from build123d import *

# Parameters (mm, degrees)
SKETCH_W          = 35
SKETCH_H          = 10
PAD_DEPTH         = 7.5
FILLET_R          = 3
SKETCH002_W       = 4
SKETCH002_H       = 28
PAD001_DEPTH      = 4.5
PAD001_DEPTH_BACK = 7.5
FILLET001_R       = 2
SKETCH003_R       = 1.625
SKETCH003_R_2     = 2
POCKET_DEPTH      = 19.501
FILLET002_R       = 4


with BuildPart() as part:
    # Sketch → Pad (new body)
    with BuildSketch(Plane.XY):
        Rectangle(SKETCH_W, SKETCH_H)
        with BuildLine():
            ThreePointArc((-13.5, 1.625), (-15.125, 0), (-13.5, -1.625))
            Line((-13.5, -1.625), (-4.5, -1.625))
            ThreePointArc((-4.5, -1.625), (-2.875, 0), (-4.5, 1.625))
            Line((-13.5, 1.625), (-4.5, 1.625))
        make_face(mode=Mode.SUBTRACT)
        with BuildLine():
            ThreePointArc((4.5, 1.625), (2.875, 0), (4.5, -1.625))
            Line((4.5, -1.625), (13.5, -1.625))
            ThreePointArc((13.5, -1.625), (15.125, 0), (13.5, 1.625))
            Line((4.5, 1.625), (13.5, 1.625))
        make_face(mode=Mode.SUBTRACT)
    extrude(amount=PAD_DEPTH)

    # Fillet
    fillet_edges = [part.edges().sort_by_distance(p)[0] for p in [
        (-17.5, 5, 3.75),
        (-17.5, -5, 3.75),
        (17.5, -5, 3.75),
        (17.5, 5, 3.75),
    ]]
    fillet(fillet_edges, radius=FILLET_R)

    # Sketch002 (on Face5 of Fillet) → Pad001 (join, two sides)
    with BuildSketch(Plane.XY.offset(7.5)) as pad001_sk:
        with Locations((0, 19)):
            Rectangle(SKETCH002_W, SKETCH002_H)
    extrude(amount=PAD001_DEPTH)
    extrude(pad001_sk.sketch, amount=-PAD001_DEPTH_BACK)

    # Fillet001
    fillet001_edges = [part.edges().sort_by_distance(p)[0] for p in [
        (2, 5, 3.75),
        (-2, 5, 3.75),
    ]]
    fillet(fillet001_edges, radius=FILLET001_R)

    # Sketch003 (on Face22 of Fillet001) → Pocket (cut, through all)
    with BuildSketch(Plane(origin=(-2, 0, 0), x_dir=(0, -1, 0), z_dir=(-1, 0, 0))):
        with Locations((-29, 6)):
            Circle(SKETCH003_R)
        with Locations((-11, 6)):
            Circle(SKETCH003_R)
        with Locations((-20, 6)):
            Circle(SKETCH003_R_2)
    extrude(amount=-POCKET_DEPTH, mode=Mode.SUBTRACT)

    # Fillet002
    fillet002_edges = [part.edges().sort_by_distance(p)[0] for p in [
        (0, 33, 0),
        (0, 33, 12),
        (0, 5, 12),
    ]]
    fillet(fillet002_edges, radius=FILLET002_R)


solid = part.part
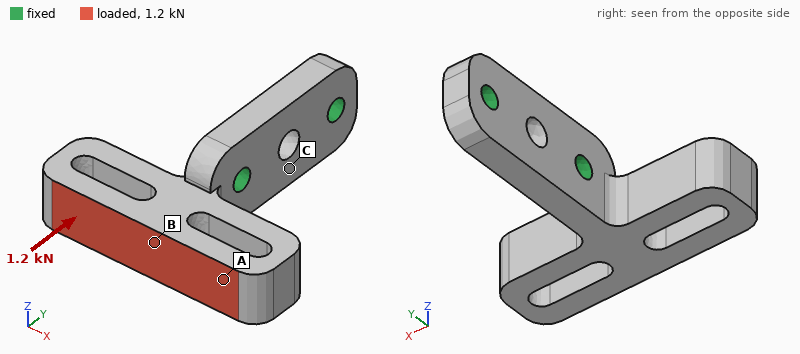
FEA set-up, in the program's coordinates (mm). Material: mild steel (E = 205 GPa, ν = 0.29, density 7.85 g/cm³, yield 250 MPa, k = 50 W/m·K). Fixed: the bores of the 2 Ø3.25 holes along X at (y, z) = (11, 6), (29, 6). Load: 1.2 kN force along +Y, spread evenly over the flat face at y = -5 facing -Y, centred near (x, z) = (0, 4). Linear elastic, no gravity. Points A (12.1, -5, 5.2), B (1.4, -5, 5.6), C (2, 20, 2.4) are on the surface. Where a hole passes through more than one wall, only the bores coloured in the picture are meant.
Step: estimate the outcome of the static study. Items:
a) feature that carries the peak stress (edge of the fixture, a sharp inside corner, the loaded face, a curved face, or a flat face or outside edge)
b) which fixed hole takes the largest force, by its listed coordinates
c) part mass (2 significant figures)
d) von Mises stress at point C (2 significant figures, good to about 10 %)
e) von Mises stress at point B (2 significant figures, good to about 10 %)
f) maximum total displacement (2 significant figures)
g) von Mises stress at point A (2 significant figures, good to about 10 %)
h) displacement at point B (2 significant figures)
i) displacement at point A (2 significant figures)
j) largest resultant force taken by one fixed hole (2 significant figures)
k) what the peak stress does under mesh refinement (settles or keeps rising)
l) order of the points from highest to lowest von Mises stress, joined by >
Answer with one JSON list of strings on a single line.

["edge of the fixture", "(11, 6)", "25 g", "11 MPa", "62 MPa", "10 µm", "28 MPa", "4.0 µm", "8.8 µm", "1.1 kN", "keeps rising", "B > A > C"]
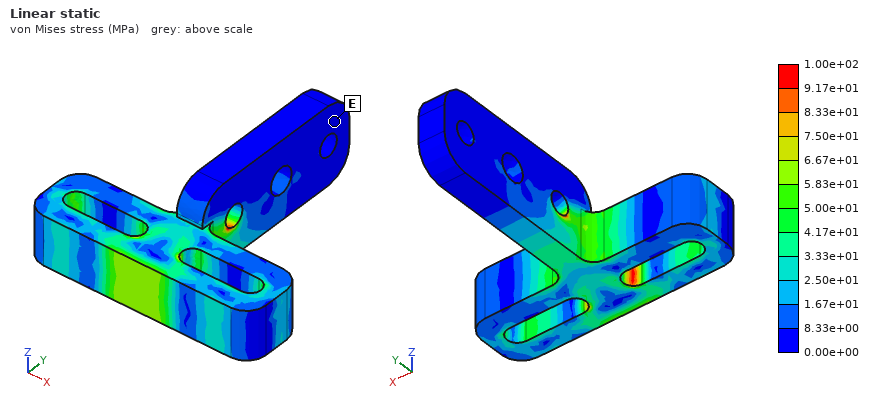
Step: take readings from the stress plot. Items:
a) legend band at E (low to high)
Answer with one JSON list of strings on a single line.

["0.00e+00 to 8.33e+00 MPa"]
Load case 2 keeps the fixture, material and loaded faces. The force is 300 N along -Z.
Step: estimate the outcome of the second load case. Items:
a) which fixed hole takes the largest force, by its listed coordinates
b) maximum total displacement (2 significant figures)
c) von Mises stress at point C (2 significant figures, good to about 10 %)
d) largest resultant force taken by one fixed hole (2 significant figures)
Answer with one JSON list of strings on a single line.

["(11, 6)", "13 µm", "15 MPa", "440 N"]
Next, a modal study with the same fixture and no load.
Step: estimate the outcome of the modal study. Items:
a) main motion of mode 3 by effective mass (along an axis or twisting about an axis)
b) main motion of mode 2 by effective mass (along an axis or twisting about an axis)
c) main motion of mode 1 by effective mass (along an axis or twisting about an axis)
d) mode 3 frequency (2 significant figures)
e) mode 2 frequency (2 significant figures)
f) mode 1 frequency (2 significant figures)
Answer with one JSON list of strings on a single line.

["along Z", "twisting about Y", "along X", "9300 Hz", "5800 Hz", "3900 Hz"]
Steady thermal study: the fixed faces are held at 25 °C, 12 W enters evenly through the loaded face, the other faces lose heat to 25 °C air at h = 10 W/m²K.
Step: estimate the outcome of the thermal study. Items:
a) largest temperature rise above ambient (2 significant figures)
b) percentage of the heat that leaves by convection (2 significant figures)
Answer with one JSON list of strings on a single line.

["72 K", "6.7 %"]
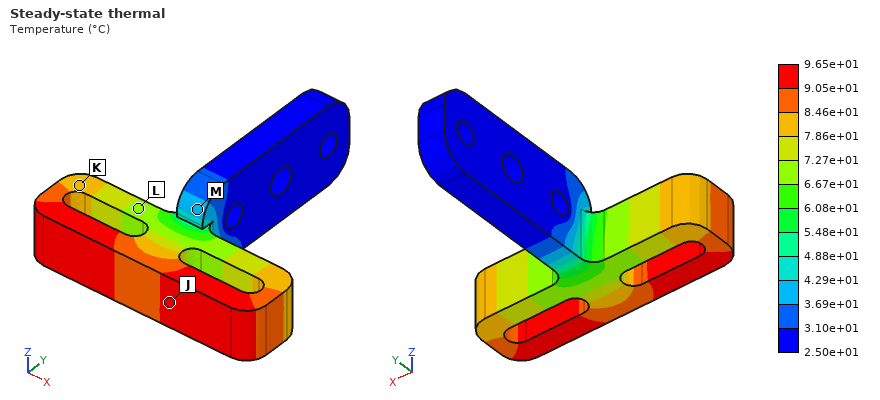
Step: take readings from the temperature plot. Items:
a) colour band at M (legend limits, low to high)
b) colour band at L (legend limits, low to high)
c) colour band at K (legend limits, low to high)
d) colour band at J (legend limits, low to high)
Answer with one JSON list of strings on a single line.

["3.69e+01 to 4.29e+01 °C", "6.67e+01 to 7.27e+01 °C", "7.86e+01 to 8.46e+01 °C", "9.05e+01 to 9.65e+01 °C"]
